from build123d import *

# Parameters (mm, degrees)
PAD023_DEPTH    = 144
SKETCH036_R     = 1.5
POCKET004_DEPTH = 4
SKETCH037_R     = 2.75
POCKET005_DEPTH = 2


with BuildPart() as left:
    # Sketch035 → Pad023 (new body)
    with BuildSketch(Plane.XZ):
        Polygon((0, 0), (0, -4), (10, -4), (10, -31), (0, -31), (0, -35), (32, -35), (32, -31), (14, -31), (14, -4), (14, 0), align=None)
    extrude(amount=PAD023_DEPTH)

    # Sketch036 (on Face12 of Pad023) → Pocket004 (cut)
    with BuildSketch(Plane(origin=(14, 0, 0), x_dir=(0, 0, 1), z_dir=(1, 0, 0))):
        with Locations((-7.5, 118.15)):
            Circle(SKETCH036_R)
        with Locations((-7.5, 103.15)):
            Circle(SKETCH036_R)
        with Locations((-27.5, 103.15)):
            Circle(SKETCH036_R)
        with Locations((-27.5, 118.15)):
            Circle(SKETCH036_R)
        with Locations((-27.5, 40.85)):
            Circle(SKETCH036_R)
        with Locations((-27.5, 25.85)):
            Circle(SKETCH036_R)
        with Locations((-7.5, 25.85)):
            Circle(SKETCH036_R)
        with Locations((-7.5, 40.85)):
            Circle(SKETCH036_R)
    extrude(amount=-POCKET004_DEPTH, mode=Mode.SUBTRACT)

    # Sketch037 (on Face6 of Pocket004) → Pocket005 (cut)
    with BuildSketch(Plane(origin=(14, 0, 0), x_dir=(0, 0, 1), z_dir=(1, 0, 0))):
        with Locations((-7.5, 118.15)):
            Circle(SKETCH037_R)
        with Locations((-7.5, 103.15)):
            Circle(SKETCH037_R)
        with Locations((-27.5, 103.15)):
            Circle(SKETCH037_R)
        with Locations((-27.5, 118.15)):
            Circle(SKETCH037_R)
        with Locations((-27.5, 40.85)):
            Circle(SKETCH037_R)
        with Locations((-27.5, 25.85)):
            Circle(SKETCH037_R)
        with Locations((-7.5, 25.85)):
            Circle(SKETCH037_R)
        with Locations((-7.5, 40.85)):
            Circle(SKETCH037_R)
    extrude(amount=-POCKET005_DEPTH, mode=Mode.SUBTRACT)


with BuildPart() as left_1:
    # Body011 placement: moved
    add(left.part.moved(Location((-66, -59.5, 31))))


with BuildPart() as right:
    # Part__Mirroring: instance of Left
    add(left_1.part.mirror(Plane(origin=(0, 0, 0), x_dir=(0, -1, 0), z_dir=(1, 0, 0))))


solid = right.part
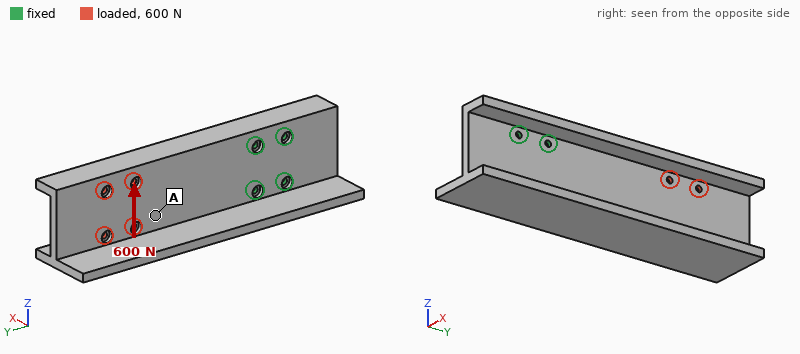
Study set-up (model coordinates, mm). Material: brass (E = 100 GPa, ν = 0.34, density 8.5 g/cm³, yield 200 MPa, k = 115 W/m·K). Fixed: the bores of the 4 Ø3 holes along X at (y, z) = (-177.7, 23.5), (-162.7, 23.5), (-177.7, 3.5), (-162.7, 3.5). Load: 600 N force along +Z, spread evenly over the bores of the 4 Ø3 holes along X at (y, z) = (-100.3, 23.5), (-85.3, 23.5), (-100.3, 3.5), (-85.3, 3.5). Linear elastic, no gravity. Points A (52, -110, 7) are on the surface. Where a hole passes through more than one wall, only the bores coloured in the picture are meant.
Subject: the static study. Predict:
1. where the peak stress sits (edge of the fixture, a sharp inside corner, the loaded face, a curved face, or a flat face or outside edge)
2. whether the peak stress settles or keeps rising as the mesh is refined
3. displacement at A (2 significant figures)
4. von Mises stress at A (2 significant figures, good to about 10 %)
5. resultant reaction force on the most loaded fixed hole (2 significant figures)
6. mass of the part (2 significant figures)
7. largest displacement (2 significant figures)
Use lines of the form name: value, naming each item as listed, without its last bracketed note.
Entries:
where the peak stress sits: edge of the fixture
whether the peak stress settles or keeps rising as the mesh is refined: keeps rising
displacement at A: 0.031 mm
von Mises stress at A: 5.4 MPa
resultant reaction force on the most loaded fixed hole: 1.2 kN
mass of the part: 350 g
largest displacement: 0.10 mm
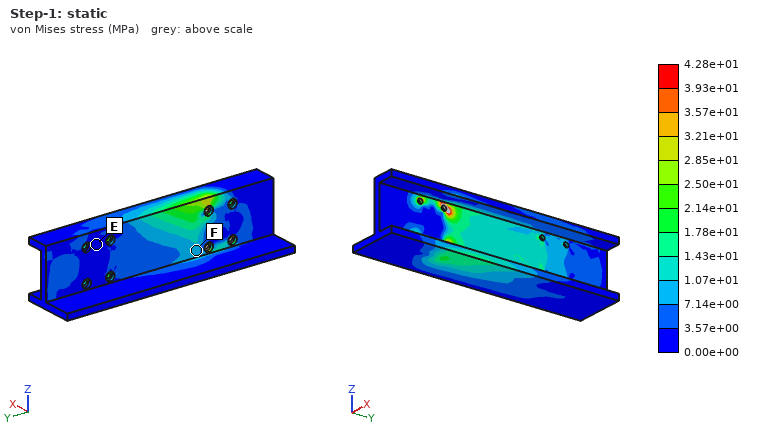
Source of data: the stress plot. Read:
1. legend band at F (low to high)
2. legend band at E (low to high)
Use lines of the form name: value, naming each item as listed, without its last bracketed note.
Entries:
legend band at F: 7.14e+00 to 1.07e+01 MPa
legend band at E: 0.00e+00 to 3.57e+00 MPa
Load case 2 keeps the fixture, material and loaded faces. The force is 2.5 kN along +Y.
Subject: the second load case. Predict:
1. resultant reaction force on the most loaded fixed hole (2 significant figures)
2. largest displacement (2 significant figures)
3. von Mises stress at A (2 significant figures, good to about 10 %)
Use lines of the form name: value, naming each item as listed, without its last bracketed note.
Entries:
resultant reaction force on the most loaded fixed hole: 860 N
largest displacement: 26 µm
von Mises stress at A: 11 MPa
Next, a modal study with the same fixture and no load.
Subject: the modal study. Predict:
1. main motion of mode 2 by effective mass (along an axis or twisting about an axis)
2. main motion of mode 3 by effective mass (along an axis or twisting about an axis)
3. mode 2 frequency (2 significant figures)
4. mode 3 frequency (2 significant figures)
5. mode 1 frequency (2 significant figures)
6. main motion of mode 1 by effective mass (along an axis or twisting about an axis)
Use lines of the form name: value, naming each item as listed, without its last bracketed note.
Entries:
main motion of mode 2 by effective mass: twisting about Y
main motion of mode 3 by effective mass: along Z
mode 2 frequency: 970 Hz
mode 3 frequency: 1400 Hz
mode 1 frequency: 590 Hz
main motion of mode 1 by effective mass: along X
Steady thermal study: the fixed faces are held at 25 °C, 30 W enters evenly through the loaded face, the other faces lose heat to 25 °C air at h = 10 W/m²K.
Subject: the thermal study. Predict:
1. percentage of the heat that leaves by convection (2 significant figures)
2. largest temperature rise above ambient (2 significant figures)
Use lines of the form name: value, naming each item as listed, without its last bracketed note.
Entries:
percentage of the heat that leaves by convection: 23 %
largest temperature rise above ambient: 66 K
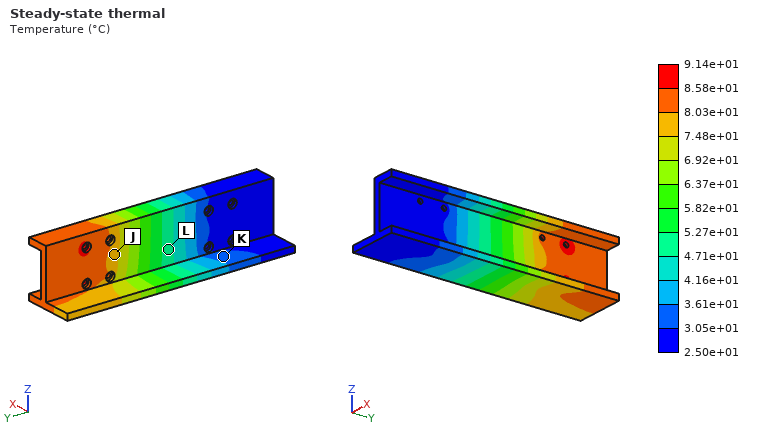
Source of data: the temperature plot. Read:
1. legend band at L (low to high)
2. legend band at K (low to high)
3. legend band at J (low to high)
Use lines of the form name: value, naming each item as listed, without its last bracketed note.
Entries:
legend band at L: 4.71e+01 to 5.27e+01 °C
legend band at K: 3.05e+01 to 3.61e+01 °C
legend band at J: 7.48e+01 to 8.03e+01 °C
